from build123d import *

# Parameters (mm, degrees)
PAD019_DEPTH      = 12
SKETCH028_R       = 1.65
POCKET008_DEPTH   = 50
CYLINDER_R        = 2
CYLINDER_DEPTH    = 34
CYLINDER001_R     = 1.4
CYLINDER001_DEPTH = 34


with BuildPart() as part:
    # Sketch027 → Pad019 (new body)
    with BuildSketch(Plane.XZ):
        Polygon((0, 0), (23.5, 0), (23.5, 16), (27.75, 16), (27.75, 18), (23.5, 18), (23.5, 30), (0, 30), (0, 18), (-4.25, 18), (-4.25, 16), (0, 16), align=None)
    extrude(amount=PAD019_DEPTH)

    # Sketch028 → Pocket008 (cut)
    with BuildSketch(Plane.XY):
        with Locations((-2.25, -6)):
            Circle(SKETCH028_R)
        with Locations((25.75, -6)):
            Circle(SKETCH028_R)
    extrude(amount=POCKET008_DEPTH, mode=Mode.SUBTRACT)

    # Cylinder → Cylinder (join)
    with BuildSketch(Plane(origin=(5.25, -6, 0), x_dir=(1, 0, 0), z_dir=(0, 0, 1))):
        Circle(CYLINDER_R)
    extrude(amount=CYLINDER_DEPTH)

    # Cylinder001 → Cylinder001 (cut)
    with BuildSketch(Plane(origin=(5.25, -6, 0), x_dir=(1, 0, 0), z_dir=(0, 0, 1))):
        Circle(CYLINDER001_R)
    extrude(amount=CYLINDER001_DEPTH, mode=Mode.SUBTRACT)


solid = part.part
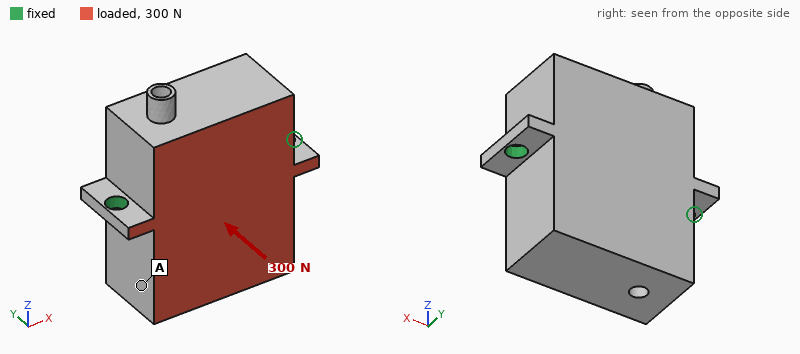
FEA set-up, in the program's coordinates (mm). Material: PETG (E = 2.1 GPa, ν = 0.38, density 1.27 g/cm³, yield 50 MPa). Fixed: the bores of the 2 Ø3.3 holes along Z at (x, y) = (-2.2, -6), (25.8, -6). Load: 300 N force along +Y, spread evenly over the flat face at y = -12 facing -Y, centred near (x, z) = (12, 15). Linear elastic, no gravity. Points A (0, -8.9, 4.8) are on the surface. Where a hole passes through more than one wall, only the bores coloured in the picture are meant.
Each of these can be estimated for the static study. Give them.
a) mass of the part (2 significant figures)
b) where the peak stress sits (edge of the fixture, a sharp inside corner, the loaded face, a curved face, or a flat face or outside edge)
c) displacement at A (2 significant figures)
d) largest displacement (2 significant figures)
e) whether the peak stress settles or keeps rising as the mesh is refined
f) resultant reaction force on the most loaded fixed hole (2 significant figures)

11 g
edge of the fixture
0.25 mm
0.35 mm
keeps rising
150 N
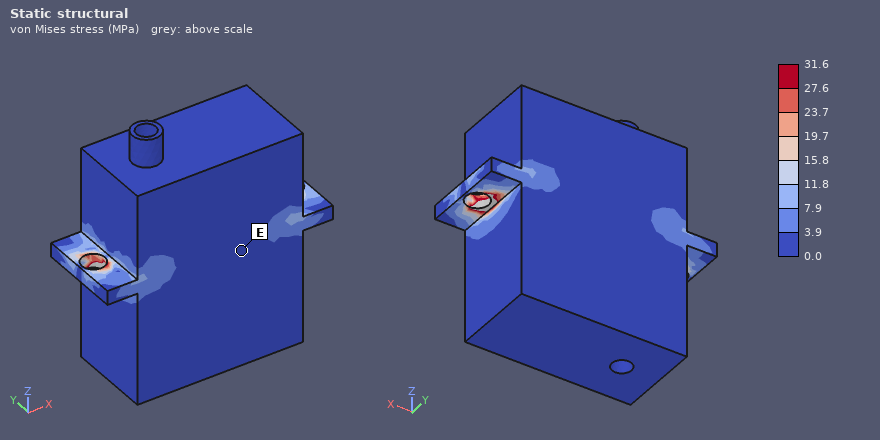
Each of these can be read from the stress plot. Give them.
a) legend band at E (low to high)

0.0 to 3.9 MPa
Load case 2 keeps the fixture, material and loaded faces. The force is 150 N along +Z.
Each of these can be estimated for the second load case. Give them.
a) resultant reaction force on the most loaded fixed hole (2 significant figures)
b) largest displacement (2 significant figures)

75 N
0.45 mm
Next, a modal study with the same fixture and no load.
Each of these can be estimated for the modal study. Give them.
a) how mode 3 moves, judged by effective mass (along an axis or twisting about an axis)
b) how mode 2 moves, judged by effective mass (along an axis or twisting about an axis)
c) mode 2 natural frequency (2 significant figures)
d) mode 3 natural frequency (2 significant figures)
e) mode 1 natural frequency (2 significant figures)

along Z
along Y
3900 Hz
4400 Hz
980 Hz
